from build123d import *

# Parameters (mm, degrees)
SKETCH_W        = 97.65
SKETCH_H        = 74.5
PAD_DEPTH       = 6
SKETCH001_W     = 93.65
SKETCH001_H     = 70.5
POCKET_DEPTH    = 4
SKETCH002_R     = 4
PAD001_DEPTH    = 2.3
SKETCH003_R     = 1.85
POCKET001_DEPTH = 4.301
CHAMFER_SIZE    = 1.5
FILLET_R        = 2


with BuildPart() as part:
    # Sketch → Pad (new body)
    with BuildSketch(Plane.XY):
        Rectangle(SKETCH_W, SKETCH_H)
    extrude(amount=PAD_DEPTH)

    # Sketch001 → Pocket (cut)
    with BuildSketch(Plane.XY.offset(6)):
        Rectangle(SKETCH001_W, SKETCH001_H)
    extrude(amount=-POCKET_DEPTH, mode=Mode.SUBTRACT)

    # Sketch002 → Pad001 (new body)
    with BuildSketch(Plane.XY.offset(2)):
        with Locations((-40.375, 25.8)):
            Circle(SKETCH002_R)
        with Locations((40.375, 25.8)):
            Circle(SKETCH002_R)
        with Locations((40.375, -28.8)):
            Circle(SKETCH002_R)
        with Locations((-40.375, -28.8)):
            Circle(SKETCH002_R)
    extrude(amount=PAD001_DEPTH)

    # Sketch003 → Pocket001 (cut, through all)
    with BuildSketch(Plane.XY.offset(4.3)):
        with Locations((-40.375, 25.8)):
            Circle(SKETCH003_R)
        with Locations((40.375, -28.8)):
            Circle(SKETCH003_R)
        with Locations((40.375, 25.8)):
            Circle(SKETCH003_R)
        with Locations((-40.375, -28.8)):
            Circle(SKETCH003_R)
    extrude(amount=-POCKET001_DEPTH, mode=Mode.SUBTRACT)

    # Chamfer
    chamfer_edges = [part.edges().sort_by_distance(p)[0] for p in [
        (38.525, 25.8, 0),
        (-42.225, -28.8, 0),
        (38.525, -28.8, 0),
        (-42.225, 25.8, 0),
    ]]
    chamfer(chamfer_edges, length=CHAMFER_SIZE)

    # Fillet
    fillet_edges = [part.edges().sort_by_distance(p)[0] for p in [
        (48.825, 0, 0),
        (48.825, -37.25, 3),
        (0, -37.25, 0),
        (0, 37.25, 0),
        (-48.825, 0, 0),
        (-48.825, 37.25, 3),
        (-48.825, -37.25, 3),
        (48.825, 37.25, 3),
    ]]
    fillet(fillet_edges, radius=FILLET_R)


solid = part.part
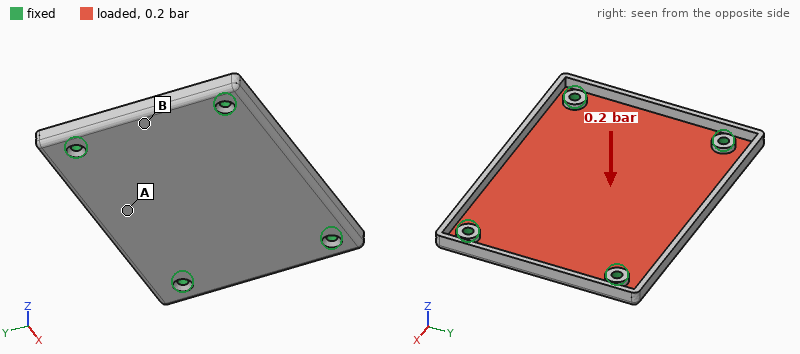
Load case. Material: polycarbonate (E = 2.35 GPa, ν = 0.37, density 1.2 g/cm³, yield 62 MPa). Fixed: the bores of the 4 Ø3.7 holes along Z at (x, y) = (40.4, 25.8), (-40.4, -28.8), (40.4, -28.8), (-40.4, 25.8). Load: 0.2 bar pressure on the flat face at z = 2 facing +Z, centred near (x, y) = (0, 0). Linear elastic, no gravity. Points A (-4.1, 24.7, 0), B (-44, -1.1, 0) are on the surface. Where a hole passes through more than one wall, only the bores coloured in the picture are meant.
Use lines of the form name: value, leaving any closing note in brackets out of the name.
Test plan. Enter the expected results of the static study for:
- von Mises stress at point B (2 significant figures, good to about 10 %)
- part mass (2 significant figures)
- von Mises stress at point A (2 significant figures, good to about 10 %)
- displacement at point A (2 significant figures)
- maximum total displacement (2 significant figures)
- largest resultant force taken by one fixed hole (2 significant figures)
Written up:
von Mises stress at point B: 2.4 MPa
part mass: 21 g
von Mises stress at point A: 4.9 MPa
displacement at point A: 0.84 mm
maximum total displacement: 1.3 mm
largest resultant force taken by one fixed hole: 43 N
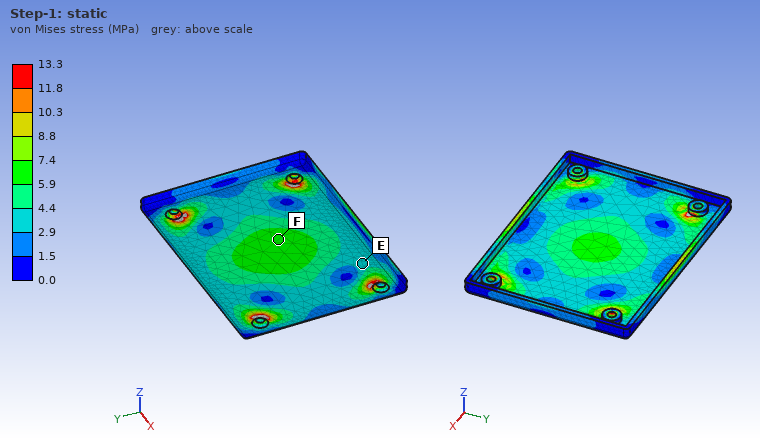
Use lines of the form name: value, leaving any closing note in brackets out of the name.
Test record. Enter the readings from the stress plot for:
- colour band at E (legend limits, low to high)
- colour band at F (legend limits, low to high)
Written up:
colour band at E: 2.9 to 4.4 MPa
colour band at F: 5.9 to 7.4 MPa
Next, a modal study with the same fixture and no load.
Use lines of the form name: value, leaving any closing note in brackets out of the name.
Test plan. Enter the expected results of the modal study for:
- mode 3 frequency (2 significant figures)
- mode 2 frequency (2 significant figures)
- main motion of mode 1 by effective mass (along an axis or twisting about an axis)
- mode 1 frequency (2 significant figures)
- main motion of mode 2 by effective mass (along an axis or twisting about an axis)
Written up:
mode 3 frequency: 970 Hz
mode 2 frequency: 750 Hz
main motion of mode 1 by effective mass: along Z
mode 1 frequency: 500 Hz
main motion of mode 2 by effective mass: twisting about X
